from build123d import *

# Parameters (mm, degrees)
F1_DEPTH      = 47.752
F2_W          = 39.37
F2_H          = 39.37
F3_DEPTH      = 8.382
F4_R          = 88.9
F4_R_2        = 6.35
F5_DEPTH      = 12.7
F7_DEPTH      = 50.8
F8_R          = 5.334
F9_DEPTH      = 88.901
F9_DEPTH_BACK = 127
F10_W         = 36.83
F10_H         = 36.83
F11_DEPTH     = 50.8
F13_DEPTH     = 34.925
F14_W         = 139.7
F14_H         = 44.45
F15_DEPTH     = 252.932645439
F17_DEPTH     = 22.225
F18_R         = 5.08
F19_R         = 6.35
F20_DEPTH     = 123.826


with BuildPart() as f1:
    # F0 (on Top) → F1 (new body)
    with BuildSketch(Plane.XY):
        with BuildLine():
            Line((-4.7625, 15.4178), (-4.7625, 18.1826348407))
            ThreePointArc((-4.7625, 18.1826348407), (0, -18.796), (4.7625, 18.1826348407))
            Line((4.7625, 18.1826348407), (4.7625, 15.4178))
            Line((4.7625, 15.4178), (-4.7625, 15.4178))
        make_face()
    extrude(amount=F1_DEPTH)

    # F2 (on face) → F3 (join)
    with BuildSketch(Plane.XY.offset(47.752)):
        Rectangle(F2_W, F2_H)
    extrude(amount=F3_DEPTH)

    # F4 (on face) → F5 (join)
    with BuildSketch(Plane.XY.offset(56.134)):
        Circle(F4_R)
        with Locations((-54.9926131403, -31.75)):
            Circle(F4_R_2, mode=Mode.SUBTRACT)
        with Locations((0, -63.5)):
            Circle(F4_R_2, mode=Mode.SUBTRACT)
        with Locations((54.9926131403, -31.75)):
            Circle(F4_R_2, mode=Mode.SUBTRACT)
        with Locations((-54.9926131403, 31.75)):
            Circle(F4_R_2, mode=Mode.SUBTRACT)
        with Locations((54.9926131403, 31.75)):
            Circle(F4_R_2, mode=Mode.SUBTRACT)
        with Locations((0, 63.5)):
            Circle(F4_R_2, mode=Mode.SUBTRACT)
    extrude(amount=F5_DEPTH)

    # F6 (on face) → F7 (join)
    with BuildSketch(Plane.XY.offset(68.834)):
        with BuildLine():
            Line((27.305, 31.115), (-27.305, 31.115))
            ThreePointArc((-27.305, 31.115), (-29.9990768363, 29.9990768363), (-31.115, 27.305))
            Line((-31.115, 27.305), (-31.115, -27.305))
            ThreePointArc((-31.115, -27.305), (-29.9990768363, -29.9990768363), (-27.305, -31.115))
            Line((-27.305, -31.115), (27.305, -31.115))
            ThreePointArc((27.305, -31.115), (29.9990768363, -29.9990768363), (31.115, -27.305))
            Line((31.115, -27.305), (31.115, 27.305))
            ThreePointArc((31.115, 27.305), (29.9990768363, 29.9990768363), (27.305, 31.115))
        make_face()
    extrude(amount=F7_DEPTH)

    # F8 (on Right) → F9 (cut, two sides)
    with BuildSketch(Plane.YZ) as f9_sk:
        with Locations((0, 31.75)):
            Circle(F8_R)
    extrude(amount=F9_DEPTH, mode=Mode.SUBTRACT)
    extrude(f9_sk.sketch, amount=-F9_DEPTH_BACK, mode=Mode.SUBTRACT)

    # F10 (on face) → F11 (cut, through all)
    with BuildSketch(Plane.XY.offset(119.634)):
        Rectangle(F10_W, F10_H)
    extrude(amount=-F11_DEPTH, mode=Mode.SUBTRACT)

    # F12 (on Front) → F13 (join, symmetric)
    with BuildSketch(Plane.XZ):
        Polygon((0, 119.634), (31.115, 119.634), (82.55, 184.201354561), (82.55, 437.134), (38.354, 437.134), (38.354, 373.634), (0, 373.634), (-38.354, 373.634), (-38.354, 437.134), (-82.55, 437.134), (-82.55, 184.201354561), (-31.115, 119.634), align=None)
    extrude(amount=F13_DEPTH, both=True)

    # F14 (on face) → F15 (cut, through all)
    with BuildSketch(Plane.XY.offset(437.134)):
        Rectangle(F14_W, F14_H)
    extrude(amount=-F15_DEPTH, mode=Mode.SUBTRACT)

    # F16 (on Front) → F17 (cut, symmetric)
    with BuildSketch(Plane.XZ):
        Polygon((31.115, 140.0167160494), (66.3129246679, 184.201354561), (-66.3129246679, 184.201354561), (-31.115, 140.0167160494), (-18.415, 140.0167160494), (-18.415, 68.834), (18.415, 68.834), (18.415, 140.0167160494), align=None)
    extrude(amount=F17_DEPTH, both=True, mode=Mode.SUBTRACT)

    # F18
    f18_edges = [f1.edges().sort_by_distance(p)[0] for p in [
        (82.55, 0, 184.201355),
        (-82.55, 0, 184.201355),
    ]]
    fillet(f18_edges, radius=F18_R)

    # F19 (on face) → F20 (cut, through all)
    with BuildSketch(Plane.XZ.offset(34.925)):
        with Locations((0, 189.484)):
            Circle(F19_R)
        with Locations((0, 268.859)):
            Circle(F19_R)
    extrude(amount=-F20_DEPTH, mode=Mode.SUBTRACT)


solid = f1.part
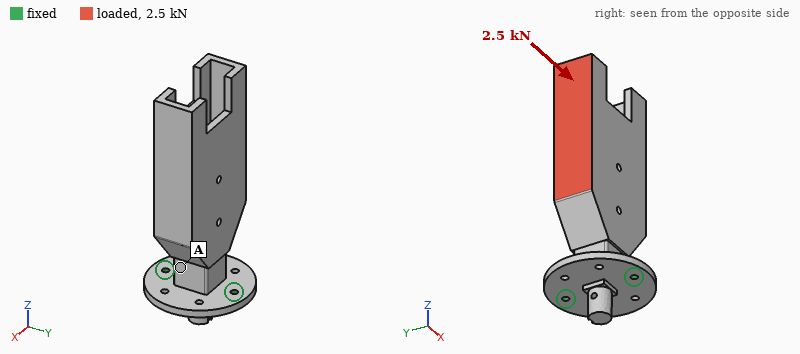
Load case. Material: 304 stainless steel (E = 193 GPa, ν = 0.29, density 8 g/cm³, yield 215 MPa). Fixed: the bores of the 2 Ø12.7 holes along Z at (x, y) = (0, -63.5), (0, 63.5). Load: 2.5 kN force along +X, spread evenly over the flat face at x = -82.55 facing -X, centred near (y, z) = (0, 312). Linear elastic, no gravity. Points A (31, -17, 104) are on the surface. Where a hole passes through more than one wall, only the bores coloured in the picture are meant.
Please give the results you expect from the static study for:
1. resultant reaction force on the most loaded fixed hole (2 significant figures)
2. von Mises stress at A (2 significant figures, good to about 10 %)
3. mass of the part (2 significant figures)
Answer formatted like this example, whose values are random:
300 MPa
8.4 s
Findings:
1.3 kN
16 MPa
16 kg
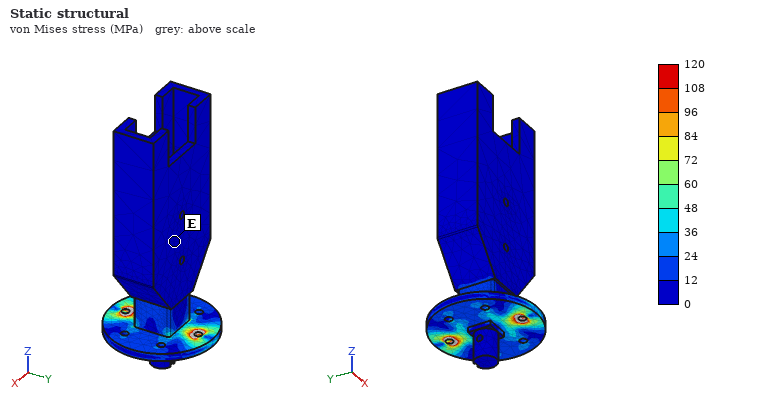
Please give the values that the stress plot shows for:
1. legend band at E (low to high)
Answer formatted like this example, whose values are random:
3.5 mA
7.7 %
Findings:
0 to 12 MPa
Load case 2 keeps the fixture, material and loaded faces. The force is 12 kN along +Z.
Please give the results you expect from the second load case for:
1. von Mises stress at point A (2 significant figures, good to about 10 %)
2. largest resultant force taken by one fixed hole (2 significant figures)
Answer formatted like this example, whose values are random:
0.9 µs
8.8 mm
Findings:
27 MPa
6.1 kN
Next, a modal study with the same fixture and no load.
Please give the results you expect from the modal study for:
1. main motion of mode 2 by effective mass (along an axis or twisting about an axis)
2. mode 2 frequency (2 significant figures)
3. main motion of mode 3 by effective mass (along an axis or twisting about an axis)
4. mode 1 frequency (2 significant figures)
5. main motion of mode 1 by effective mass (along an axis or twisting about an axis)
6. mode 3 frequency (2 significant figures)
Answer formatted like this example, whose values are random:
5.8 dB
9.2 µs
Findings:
along Y
200 Hz
twisting about Z
100 Hz
along X
750 Hz
